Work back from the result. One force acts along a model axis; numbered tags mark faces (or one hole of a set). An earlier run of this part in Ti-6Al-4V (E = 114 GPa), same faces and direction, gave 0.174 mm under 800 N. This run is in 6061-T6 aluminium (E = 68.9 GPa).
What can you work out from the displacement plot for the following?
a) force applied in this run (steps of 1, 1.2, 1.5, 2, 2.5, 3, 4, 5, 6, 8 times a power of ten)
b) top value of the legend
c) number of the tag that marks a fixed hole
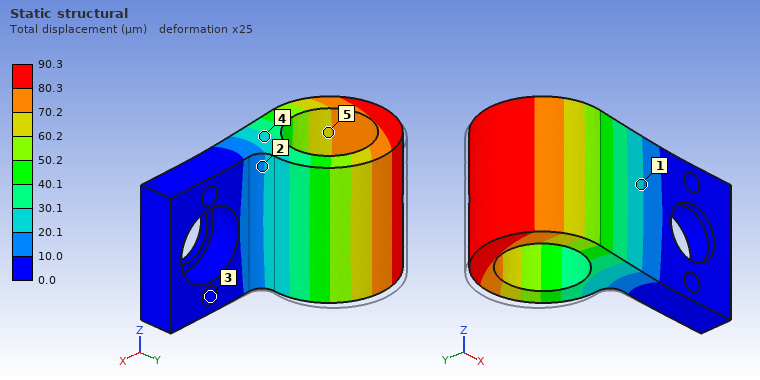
250 N
90.3 µm
3
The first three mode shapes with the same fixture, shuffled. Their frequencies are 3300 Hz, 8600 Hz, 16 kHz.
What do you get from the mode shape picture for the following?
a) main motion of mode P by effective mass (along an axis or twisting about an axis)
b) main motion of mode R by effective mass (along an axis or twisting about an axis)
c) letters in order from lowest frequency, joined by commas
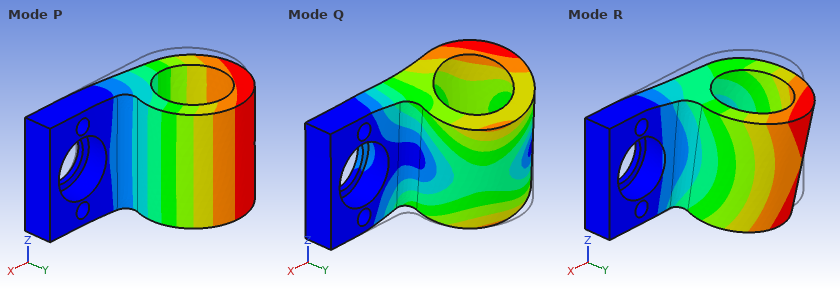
along Y
along Z
P, R, Q
